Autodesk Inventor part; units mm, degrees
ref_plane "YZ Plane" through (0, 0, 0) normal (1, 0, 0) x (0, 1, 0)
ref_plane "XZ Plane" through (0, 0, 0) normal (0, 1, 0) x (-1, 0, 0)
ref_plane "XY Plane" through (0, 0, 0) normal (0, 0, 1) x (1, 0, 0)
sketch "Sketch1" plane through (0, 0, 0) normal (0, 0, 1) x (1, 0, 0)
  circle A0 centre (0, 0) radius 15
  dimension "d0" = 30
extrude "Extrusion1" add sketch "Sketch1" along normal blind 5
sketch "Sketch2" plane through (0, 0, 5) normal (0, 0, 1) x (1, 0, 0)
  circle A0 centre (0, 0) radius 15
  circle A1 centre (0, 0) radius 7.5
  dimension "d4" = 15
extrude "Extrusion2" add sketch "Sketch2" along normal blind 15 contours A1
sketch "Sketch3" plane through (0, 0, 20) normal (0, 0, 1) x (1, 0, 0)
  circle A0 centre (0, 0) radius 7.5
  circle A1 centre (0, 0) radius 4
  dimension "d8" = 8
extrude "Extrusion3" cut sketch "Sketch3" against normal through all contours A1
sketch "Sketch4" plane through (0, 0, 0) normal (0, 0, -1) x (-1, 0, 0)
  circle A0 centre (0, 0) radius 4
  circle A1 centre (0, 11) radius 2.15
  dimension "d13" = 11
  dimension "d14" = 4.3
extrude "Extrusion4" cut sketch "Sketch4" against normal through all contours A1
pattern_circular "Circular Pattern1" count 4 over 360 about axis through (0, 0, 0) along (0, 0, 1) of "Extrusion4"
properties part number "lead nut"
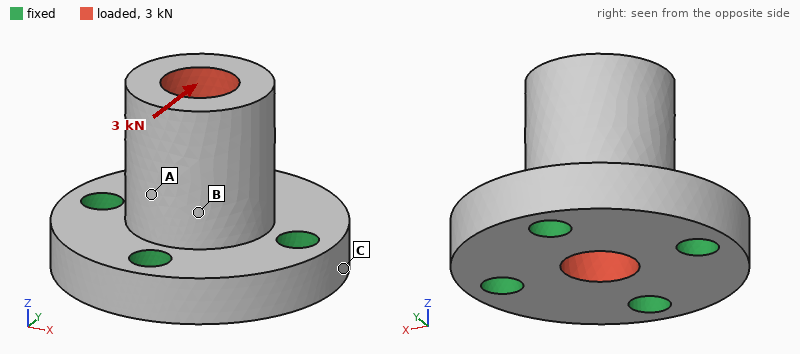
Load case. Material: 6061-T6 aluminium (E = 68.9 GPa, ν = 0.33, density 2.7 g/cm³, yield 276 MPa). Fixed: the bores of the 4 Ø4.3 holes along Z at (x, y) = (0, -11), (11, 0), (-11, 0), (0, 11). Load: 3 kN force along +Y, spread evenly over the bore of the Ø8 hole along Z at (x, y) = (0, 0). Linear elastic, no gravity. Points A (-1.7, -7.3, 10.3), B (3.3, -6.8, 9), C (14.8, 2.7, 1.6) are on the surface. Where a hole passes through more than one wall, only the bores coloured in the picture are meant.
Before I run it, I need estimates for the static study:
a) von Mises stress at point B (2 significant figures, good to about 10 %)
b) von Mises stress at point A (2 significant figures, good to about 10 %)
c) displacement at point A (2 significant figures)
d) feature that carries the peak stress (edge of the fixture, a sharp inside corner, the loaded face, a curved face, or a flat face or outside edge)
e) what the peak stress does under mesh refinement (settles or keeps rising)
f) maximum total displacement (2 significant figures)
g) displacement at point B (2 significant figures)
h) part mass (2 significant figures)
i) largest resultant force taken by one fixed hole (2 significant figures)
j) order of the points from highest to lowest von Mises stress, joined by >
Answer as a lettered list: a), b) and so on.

a) 28 MPa
b) 20 MPa
c) 13 µm
d) a sharp inside corner
e) keeps rising
f) 26 µm
g) 11 µm
h) 13 g
i) 1.5 kN
j) B > A > C
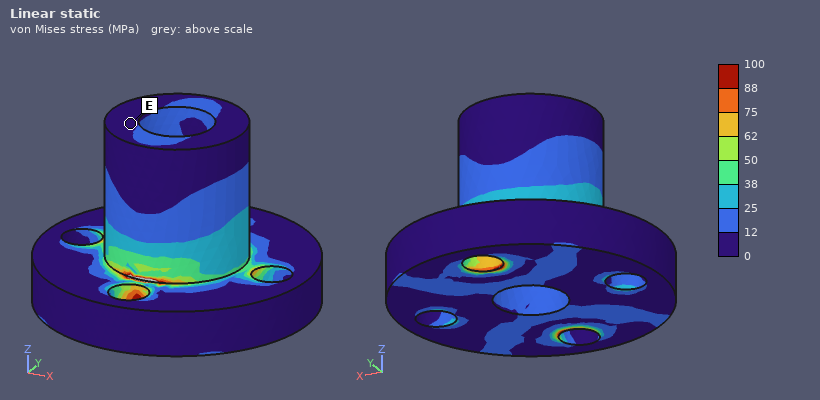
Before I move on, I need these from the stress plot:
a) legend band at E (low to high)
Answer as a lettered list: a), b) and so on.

a) 0 to 12 MPa
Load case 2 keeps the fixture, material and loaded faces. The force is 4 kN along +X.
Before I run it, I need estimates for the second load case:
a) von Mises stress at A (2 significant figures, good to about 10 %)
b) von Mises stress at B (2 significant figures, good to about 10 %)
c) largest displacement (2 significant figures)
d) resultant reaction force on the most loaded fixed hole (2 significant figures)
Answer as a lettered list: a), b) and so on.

a) 35 MPa
b) 37 MPa
c) 35 µm
d) 2.0 kN
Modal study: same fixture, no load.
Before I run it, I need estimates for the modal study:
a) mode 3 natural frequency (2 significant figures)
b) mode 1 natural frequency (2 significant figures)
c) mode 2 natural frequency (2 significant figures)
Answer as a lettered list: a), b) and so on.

a) 46 kHz
b) 24 kHz
c) 24 kHz
